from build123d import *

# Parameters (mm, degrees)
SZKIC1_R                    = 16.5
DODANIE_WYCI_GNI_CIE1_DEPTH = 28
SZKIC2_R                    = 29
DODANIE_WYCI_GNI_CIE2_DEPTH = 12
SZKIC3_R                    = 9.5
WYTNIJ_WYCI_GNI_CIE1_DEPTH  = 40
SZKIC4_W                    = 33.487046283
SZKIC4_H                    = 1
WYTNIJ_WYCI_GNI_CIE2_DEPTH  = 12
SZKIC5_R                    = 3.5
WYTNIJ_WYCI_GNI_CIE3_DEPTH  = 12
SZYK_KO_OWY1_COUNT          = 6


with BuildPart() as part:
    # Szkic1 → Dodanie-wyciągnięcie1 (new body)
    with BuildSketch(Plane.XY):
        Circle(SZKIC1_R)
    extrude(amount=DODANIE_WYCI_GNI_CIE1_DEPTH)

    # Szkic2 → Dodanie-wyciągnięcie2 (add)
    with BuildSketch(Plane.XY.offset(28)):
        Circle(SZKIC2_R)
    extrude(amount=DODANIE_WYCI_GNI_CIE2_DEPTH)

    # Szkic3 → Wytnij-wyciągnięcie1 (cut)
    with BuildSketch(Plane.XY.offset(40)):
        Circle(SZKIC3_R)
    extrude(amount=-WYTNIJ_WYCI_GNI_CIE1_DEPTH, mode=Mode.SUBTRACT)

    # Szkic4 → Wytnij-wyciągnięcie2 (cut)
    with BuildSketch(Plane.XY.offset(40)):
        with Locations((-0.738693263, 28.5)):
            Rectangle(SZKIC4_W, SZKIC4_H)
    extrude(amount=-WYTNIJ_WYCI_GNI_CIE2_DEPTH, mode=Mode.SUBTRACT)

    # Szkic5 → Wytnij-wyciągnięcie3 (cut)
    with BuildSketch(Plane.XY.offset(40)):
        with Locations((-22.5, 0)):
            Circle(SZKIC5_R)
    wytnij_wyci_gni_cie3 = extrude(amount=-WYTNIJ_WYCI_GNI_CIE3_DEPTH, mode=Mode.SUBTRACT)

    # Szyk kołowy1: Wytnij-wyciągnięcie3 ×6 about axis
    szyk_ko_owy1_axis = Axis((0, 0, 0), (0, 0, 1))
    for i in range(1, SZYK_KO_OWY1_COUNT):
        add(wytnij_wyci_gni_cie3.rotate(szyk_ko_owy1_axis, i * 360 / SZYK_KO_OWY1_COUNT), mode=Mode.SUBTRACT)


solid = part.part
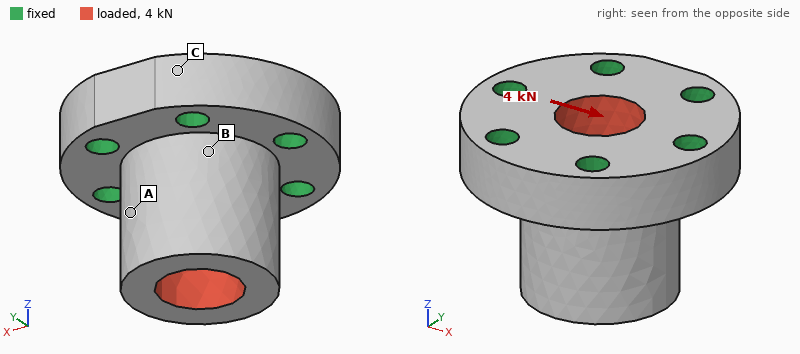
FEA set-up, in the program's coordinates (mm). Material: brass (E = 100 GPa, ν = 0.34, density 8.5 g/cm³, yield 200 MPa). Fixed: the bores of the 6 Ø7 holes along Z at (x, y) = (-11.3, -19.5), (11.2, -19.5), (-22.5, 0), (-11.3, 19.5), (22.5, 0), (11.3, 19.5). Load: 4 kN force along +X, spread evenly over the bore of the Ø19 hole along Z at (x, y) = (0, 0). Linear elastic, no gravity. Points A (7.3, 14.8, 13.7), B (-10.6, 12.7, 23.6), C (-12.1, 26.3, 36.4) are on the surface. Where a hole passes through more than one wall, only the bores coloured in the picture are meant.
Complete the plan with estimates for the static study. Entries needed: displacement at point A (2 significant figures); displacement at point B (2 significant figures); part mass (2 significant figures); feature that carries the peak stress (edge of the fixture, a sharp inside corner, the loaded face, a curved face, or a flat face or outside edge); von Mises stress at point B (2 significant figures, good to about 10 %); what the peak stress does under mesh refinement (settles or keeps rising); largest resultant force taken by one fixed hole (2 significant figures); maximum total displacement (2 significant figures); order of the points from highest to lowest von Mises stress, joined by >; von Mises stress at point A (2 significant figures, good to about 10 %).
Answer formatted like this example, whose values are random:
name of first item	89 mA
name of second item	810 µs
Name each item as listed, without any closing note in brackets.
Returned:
displacement at point A	4.0 µm
displacement at point B	2.0 µm
part mass	350 g
feature that carries the peak stress	a sharp inside corner
von Mises stress at point B	8.7 MPa
what the peak stress does under mesh refinement	keeps rising
largest resultant force taken by one fixed hole	1.3 kN
maximum total displacement	7.2 µm
order of the points from highest to lowest von Mises stress, joined by >	B > A > C
von Mises stress at point A	5.6 MPa
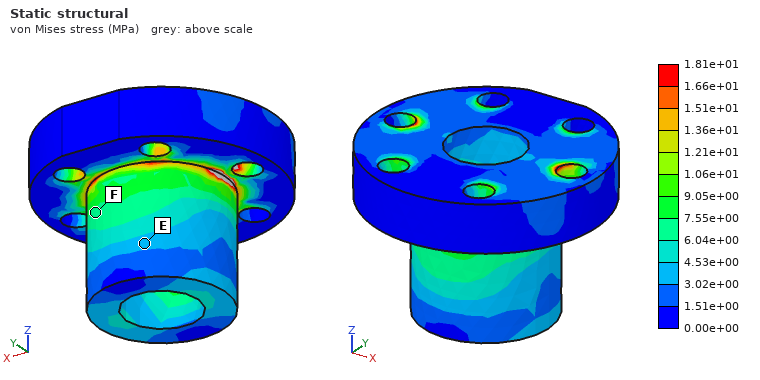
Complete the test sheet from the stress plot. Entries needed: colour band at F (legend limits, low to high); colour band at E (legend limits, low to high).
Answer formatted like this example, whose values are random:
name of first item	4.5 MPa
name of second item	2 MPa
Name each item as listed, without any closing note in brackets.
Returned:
colour band at F	6.04e+00 to 7.55e+00 MPa
colour band at E	3.02e+00 to 4.53e+00 MPa
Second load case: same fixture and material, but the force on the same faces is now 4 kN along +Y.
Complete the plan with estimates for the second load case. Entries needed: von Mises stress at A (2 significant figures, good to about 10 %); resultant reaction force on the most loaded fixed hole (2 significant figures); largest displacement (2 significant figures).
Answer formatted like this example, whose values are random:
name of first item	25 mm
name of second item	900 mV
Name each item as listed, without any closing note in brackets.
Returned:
von Mises stress at A	3.8 MPa
resultant reaction force on the most loaded fixed hole	1.2 kN
largest displacement	7.2 µm
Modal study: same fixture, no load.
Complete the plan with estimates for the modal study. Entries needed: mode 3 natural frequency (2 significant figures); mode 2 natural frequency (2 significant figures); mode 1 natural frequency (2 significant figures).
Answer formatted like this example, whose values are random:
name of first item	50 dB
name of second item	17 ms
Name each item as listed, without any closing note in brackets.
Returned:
mode 3 natural frequency	16 kHz
mode 2 natural frequency	10 kHz
mode 1 natural frequency	10 kHz
